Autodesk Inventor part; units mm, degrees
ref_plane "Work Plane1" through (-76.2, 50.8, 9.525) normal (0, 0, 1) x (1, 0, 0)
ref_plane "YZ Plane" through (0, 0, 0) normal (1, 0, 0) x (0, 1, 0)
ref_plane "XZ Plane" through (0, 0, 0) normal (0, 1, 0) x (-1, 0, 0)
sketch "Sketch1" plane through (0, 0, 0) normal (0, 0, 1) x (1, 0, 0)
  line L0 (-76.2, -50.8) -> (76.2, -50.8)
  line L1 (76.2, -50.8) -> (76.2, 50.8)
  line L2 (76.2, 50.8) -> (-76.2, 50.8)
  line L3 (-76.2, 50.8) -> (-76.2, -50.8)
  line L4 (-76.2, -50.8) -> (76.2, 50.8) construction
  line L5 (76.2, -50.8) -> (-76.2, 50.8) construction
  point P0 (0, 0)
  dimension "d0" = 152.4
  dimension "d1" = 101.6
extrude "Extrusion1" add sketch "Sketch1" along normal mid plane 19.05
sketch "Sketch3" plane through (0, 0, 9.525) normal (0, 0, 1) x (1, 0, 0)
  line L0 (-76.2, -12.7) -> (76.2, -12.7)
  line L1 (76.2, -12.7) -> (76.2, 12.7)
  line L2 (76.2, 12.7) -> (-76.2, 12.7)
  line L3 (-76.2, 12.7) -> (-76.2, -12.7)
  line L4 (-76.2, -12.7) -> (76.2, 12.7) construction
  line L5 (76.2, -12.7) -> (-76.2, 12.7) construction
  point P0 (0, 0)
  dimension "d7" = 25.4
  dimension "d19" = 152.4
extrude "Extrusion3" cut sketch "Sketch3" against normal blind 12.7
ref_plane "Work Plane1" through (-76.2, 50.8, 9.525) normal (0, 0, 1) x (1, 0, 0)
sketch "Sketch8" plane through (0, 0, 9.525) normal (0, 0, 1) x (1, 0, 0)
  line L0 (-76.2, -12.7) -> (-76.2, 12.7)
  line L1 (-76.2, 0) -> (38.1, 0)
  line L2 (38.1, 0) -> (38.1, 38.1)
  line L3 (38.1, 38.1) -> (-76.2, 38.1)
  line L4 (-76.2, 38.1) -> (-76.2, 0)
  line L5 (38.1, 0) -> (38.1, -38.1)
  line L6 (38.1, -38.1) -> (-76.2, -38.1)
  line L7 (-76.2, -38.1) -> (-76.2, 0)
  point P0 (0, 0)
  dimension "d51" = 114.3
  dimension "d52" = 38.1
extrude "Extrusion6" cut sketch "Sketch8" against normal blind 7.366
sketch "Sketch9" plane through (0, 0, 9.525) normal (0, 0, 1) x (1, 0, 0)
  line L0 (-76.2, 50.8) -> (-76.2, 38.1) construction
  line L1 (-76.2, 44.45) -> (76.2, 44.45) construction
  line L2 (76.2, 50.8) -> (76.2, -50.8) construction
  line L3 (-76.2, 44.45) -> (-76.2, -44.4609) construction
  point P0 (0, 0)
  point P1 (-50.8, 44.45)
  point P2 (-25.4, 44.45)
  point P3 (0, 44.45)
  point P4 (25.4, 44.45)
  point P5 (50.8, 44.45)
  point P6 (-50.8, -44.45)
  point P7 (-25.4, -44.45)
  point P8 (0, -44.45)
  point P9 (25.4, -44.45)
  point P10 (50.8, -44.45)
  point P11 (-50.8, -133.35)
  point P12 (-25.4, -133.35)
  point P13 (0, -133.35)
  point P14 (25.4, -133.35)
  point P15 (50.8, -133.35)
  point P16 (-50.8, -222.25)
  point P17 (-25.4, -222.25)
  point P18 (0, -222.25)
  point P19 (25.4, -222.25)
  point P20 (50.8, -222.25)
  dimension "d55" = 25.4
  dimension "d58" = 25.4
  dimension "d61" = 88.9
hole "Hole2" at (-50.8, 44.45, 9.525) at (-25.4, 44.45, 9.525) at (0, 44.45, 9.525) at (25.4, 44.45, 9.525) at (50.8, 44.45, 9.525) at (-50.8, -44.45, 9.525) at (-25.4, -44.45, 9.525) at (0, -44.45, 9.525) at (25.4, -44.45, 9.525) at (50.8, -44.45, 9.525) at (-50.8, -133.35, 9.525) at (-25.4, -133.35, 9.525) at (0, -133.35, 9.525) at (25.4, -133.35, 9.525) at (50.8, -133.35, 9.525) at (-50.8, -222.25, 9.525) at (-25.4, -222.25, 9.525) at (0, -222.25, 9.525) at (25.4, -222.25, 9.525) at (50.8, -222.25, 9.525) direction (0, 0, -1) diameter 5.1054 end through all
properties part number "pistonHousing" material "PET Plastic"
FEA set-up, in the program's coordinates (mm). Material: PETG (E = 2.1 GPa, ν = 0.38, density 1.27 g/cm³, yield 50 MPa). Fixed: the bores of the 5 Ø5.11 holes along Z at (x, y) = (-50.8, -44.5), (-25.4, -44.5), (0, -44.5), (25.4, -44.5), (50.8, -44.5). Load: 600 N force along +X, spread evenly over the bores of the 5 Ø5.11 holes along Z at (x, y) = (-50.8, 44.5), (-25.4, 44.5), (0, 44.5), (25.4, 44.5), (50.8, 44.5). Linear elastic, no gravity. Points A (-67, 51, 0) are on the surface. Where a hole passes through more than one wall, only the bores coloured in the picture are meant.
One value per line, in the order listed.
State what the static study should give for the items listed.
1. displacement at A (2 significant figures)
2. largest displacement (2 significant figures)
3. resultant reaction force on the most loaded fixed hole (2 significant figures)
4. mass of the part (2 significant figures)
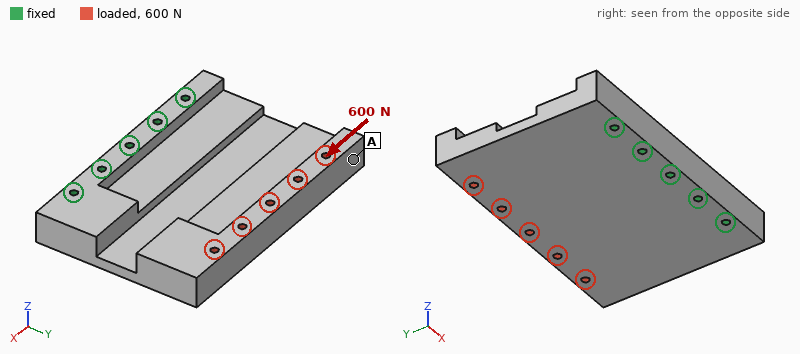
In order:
0.27 mm
0.31 mm
480 N
250 g
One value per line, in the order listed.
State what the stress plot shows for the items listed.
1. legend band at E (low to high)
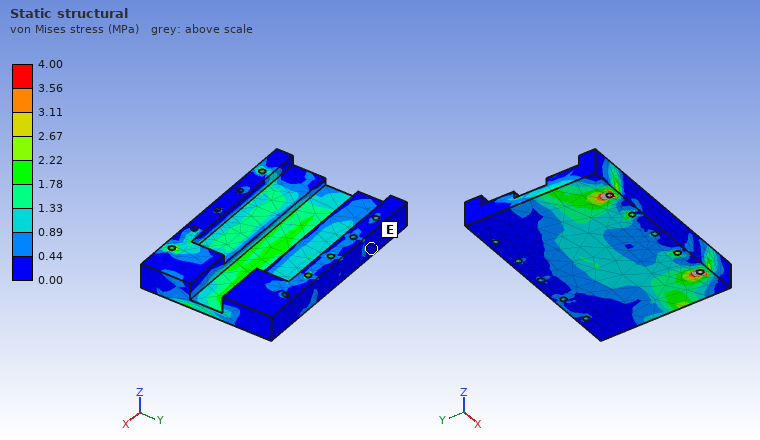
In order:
0.00 to 0.44 MPa
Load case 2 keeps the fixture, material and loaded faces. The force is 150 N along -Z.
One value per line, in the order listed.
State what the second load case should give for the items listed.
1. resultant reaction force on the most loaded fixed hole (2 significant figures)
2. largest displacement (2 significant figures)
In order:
49 N
1.9 mm
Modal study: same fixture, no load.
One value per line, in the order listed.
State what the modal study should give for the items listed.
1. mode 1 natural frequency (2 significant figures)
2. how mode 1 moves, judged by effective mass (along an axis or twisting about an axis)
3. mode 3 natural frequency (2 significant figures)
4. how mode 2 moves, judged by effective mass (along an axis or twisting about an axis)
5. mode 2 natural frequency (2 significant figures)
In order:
180 Hz
along Z
990 Hz
twisting about Y
370 Hz
